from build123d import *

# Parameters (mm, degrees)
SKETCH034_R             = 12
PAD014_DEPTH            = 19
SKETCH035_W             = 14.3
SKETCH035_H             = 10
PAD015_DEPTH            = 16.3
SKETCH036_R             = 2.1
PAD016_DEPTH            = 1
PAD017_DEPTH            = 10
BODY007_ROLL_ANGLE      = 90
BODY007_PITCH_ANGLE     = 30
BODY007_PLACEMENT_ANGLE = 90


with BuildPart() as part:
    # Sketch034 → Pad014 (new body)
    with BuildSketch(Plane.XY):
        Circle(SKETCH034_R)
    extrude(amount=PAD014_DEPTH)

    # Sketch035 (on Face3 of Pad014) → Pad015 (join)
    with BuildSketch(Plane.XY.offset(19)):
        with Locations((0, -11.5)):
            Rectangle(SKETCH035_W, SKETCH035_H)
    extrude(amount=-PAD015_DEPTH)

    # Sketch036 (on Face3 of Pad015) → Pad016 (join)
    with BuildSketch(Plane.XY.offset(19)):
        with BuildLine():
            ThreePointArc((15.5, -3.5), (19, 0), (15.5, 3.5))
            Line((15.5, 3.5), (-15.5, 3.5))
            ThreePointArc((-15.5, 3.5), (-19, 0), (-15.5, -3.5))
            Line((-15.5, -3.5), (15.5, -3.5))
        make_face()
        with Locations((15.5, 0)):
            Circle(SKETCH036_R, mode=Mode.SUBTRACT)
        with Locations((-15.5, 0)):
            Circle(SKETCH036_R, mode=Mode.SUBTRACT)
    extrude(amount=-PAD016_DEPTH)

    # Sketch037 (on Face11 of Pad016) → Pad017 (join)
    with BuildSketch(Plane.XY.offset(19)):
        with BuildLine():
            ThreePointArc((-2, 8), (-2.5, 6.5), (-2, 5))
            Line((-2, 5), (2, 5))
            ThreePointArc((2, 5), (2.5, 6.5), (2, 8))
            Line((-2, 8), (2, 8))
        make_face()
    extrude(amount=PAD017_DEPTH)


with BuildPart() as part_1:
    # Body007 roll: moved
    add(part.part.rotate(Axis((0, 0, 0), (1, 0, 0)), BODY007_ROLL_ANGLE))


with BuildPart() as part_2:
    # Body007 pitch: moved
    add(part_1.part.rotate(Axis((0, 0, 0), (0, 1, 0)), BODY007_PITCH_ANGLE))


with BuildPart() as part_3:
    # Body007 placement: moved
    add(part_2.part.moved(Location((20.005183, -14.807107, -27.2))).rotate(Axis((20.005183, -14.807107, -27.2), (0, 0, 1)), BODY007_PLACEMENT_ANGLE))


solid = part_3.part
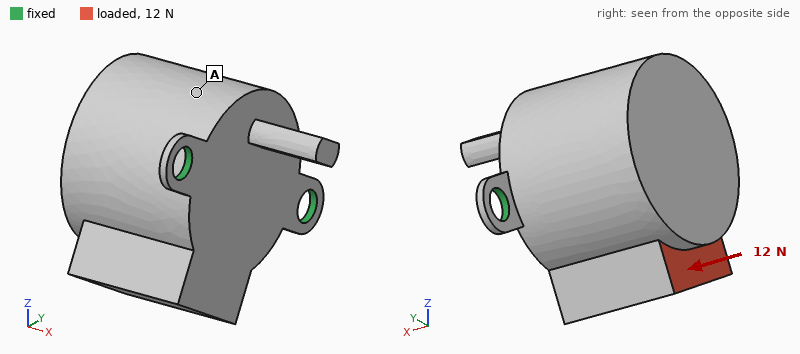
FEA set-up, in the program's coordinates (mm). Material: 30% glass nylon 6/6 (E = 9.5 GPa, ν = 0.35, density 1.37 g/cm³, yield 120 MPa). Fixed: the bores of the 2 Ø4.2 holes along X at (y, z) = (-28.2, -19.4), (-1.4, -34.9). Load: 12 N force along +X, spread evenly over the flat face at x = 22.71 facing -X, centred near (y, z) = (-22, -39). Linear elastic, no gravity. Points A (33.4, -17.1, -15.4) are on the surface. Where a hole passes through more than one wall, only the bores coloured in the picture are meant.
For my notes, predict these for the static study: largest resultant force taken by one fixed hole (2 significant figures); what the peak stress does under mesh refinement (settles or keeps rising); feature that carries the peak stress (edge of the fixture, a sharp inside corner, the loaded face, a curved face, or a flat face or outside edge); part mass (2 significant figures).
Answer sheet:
7.2 N
keeps rising
edge of the fixture
14 g
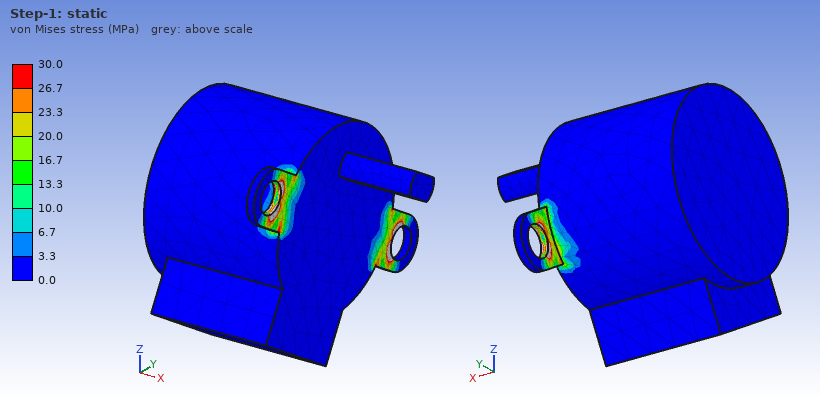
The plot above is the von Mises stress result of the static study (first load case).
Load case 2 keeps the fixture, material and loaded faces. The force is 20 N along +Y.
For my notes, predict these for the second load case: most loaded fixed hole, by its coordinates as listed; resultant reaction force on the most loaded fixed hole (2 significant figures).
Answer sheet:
(-1.4, -34.9)
20 N
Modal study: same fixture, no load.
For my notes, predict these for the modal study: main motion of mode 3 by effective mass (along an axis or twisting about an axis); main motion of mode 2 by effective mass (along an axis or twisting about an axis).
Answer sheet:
along Y
along X
